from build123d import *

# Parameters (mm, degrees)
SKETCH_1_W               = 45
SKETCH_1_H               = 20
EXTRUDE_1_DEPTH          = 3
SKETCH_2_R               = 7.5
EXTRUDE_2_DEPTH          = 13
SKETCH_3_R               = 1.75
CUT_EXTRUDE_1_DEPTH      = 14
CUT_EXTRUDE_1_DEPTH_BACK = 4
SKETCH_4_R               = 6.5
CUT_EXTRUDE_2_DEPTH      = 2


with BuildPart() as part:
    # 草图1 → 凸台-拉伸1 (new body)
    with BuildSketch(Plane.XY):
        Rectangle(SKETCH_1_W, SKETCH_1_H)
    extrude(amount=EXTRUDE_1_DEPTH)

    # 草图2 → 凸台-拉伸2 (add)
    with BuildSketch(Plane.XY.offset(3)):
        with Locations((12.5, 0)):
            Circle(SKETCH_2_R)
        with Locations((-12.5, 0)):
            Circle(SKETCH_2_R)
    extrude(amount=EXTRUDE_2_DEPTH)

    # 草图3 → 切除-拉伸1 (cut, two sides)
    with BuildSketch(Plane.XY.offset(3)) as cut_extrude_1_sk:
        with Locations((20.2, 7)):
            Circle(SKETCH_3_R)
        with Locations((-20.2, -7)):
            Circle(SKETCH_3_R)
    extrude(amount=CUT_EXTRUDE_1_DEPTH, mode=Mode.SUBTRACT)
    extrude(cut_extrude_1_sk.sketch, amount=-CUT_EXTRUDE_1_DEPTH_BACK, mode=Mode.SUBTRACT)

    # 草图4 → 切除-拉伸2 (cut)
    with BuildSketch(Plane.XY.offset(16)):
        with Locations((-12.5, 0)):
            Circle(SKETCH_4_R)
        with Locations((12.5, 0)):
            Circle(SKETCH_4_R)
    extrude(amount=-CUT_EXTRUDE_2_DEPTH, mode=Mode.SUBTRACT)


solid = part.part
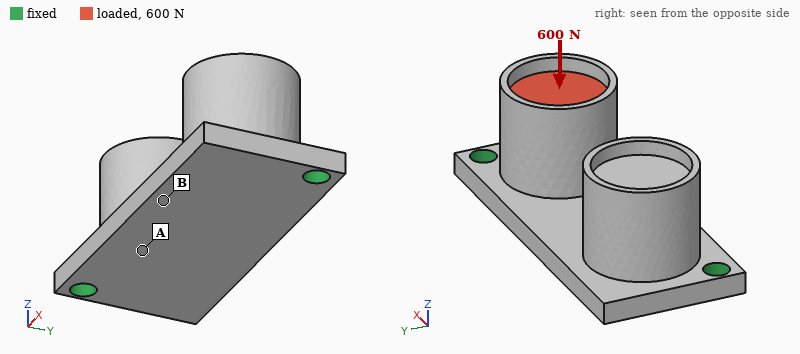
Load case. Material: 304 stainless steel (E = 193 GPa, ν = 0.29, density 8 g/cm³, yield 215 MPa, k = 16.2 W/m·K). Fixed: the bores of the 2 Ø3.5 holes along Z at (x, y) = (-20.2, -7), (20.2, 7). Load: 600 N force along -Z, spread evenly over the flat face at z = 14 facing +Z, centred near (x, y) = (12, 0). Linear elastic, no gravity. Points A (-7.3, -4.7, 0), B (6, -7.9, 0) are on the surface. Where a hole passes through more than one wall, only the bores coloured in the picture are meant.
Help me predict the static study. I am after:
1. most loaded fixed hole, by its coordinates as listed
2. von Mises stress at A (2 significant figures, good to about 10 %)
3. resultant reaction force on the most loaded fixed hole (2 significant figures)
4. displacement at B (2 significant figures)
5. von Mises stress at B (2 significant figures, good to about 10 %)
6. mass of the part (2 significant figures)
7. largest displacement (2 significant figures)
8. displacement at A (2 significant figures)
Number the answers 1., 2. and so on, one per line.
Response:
1. (20.2, 7)
2. 23 MPa
3. 490 N
4. 22 µm
5. 52 MPa
6. 54 g
7. 28 µm
8. 9.6 µm
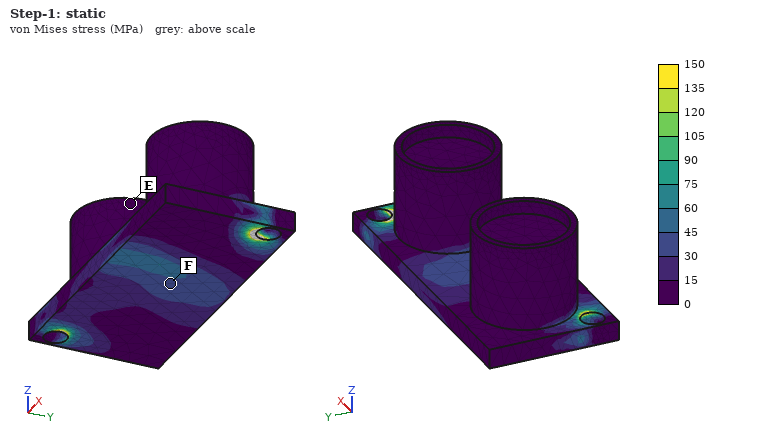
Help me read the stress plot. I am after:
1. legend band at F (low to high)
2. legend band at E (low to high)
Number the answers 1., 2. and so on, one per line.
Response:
1. 30 to 45 MPa
2. 0 to 15 MPa
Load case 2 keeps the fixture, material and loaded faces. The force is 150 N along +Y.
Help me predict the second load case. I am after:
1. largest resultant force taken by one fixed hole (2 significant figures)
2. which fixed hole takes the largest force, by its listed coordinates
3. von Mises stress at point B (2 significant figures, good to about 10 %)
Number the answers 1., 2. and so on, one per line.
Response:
1. 130 N
2. (20.2, 7)
3. 15 MPa
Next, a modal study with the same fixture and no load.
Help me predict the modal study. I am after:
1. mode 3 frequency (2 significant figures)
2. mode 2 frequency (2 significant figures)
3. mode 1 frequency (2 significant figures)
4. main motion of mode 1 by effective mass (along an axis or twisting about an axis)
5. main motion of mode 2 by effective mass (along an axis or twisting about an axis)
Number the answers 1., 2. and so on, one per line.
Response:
1. 7800 Hz
2. 4800 Hz
3. 4400 Hz
4. along Z
5. along Y
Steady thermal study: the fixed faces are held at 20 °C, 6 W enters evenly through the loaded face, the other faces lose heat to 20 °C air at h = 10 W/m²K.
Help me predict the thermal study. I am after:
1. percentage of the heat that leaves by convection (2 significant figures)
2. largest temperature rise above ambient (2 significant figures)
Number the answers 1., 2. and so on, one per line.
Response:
1. 15 %
2. 64 K
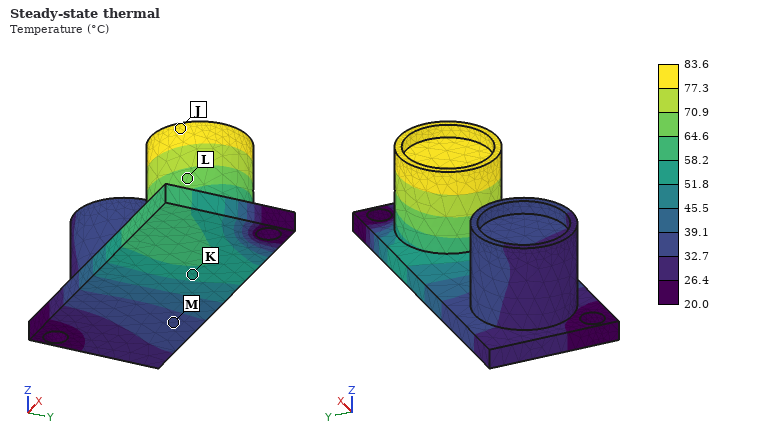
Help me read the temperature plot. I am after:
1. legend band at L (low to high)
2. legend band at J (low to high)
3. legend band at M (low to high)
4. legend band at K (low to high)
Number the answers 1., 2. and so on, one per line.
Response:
1. 64.6 to 70.9 °C
2. 77.3 to 83.6 °C
3. 32.7 to 39.1 °C
4. 51.8 to 58.2 °C
